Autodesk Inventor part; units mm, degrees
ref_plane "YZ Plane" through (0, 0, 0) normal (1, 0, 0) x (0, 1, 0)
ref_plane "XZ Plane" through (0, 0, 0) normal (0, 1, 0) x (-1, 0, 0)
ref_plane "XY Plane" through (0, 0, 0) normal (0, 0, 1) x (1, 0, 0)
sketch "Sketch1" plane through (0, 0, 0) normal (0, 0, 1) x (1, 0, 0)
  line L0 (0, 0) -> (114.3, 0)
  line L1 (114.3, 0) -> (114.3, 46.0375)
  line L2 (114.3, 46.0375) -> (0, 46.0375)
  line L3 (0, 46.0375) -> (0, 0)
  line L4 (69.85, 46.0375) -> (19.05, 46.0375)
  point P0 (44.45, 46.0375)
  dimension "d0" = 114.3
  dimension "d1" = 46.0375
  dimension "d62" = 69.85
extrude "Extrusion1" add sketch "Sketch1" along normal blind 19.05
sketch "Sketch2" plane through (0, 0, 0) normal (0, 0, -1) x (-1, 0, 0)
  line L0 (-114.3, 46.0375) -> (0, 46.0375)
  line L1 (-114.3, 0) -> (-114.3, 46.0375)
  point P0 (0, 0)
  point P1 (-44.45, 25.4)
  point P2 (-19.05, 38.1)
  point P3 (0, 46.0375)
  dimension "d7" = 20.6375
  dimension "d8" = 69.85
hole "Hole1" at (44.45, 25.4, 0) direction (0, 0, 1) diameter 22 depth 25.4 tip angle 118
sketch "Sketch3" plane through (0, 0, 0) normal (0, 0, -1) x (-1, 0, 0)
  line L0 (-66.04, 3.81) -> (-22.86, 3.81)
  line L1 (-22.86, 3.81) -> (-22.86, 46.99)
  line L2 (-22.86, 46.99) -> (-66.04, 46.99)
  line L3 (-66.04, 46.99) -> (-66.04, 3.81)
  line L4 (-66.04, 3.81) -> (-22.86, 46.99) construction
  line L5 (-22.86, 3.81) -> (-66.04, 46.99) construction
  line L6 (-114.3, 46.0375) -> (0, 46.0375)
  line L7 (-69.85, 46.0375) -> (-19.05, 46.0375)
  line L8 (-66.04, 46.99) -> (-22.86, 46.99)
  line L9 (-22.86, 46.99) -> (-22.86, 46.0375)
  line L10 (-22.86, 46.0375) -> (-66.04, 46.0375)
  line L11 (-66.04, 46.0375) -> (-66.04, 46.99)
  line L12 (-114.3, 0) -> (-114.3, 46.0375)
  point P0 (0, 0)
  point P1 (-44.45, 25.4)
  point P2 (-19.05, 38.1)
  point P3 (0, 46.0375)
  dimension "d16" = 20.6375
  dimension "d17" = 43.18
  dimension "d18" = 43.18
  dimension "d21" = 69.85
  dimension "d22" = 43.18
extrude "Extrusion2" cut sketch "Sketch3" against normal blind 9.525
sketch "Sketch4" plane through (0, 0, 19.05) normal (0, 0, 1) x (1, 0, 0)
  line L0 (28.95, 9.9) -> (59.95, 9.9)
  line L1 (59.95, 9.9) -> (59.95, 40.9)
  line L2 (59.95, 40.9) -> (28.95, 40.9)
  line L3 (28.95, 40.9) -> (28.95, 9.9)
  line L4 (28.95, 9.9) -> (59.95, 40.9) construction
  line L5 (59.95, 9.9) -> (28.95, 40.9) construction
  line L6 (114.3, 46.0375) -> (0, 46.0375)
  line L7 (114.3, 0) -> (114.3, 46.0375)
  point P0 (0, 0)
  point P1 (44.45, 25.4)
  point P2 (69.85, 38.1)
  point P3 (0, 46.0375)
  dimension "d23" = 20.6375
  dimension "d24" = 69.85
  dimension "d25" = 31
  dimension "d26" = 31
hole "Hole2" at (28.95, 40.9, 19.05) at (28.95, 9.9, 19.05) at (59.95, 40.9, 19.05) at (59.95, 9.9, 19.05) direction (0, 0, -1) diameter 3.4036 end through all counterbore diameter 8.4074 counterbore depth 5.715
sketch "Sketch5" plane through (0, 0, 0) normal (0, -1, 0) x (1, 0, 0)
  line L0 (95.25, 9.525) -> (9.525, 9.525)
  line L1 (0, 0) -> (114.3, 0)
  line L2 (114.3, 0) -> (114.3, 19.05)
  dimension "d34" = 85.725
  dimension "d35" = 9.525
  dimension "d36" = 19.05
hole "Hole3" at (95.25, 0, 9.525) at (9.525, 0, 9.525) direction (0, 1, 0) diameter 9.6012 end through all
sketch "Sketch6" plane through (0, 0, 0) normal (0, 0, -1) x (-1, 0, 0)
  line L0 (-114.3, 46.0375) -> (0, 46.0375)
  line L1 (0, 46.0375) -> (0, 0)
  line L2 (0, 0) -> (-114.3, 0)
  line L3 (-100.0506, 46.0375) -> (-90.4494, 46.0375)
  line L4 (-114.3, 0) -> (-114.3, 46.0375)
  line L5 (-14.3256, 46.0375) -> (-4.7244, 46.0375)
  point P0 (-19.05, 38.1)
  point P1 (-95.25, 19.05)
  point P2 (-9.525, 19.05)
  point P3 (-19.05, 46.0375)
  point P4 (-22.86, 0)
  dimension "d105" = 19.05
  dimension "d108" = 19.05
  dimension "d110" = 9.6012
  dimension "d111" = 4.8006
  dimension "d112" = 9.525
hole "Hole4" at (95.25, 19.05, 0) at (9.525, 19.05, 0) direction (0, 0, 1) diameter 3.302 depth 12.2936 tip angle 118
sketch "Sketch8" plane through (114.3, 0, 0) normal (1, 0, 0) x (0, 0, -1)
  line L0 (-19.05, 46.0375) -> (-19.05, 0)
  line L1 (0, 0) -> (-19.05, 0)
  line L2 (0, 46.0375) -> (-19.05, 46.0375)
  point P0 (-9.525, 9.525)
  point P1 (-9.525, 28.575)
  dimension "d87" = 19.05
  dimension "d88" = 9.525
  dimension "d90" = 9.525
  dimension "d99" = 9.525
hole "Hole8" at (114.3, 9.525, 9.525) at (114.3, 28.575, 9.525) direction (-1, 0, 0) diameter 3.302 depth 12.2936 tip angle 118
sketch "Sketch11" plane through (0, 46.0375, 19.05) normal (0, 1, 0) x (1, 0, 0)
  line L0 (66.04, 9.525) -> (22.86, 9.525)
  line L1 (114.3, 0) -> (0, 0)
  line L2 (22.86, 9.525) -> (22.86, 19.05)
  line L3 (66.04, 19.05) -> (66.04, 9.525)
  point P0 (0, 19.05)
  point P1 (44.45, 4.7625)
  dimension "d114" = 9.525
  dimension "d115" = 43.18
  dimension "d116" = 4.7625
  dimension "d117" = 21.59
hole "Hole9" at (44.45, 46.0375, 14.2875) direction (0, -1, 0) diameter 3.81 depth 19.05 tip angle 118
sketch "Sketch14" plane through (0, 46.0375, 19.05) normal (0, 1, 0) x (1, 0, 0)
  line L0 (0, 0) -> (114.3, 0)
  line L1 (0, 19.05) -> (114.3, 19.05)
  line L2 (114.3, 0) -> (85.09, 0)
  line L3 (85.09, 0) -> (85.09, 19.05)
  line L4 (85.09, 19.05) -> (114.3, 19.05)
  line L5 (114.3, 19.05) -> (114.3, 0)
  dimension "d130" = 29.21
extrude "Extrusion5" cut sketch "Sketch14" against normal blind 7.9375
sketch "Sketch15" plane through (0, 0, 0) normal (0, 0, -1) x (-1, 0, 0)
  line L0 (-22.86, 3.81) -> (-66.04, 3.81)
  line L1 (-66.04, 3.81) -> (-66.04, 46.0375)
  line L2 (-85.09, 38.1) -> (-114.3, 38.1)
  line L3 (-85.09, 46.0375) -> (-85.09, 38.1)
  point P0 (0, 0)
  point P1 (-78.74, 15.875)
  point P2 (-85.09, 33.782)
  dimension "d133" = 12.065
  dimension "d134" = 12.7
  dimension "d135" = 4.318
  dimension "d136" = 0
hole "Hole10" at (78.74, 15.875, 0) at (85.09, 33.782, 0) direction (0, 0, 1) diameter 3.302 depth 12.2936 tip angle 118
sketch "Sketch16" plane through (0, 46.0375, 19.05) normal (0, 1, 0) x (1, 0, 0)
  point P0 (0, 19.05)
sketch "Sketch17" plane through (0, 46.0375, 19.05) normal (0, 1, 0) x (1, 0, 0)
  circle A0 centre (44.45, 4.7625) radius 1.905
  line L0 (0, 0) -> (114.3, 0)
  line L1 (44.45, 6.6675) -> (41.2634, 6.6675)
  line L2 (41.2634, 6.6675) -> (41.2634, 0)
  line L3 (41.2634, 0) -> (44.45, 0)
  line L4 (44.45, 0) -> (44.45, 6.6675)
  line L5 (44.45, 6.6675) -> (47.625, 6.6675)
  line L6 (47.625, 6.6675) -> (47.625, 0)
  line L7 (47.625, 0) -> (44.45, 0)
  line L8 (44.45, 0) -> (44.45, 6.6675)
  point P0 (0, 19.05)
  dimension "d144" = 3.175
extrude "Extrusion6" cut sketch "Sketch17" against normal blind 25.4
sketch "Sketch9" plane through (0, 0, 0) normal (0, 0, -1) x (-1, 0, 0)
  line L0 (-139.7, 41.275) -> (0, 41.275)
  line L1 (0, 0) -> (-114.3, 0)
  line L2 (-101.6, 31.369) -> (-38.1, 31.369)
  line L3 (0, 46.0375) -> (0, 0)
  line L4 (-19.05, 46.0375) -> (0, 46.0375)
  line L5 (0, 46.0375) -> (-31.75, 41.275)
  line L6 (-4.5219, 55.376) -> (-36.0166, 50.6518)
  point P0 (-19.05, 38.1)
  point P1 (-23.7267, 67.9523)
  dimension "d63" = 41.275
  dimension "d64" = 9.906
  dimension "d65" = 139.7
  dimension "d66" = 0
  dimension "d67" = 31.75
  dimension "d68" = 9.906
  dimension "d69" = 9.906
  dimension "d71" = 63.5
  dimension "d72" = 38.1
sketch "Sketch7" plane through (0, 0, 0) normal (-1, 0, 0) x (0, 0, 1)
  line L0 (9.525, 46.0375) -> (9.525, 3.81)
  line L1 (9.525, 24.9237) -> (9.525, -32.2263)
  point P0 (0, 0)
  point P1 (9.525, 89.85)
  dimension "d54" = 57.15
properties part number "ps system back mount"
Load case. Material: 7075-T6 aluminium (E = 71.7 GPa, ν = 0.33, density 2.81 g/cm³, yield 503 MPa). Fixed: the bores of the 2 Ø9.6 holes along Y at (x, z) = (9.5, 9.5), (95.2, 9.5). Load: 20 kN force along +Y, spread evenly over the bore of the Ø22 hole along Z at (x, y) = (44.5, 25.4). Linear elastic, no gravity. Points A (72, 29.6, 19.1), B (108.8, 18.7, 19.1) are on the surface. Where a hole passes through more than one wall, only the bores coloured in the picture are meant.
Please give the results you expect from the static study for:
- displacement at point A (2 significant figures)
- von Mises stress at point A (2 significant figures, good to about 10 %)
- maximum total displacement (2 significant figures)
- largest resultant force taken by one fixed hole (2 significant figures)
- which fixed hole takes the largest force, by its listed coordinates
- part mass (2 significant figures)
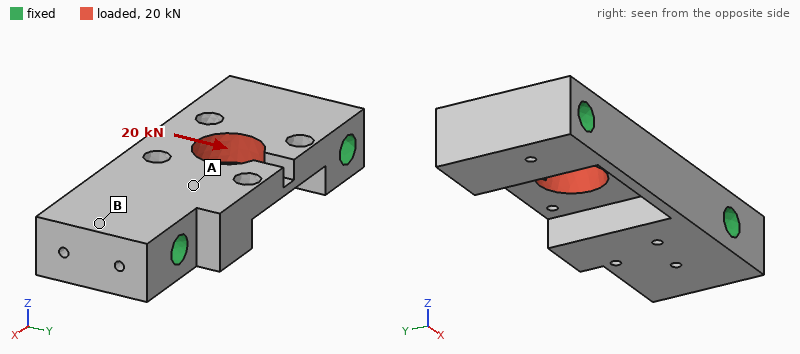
20 µm
30 MPa
65 µm
12 kN
(9.5, 9.5)
190 g
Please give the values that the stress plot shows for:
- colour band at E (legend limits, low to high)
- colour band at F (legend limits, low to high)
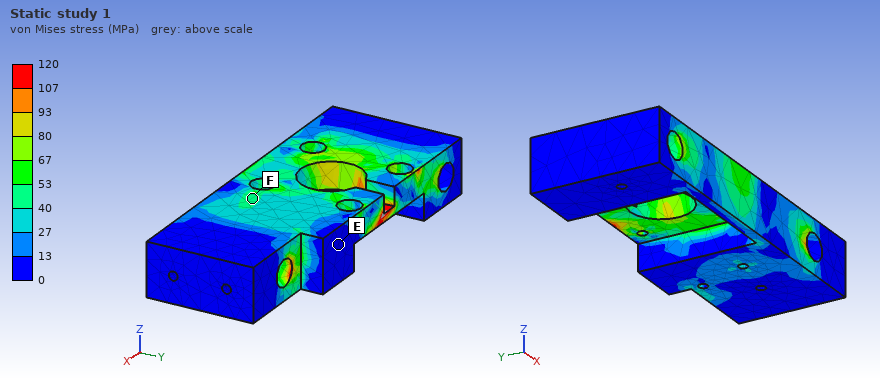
0 to 13 MPa
40 to 53 MPa
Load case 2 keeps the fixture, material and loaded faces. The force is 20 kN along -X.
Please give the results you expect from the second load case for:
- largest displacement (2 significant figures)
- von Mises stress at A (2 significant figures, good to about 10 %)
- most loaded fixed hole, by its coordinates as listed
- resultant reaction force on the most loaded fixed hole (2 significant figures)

20 µm
29 MPa
(9.5, 9.5)
11 kN
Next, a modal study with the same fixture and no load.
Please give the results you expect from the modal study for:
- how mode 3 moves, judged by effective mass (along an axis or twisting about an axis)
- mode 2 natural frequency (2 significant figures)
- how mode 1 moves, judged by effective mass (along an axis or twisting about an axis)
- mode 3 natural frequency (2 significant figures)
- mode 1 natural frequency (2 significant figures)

along Y
13 kHz
along Z
15 kHz
9600 Hz
